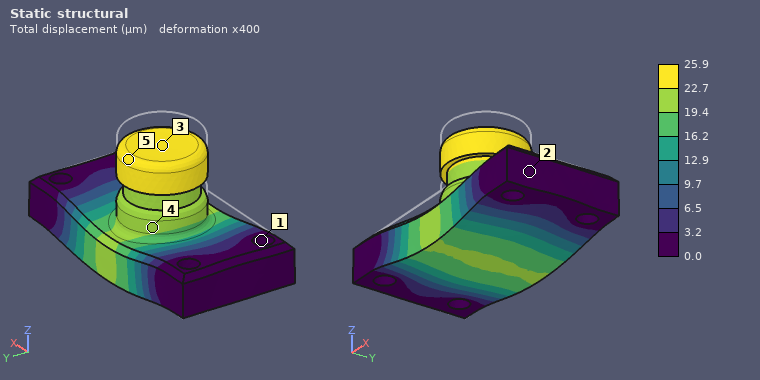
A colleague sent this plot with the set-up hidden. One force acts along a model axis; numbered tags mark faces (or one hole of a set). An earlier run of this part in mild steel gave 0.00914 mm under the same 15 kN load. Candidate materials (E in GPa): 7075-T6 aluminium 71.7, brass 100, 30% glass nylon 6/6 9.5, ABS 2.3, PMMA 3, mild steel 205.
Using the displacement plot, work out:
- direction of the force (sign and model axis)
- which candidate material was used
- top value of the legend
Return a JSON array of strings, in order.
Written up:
["-Z", "7075-T6 aluminium", "25.9 µm"]
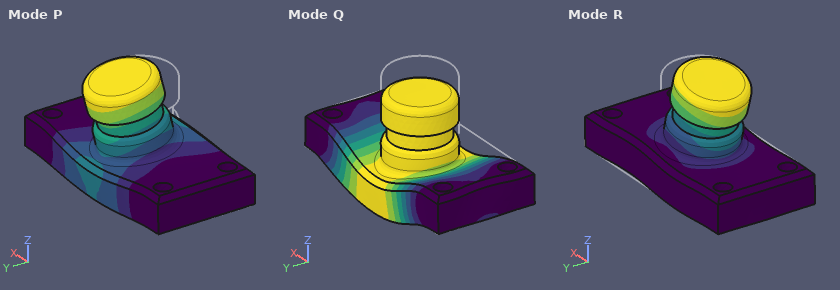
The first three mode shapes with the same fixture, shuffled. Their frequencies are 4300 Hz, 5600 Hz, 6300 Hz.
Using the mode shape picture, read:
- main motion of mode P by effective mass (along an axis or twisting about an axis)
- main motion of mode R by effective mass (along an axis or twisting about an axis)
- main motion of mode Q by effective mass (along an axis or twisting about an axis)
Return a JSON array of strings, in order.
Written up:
["along Y", "along X", "along Z"]
